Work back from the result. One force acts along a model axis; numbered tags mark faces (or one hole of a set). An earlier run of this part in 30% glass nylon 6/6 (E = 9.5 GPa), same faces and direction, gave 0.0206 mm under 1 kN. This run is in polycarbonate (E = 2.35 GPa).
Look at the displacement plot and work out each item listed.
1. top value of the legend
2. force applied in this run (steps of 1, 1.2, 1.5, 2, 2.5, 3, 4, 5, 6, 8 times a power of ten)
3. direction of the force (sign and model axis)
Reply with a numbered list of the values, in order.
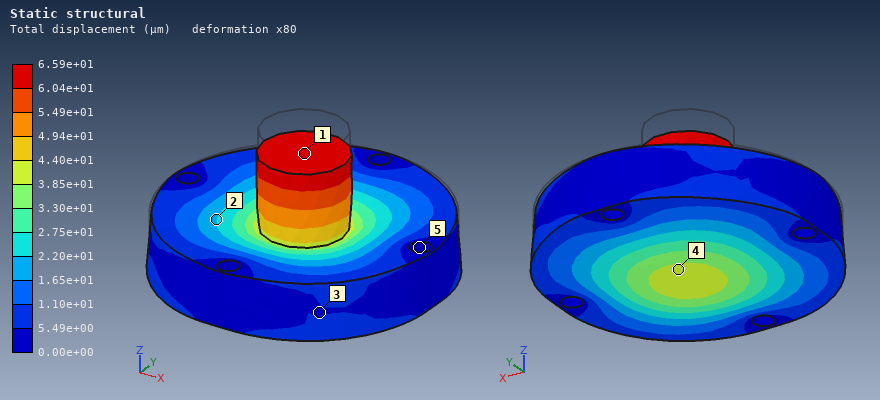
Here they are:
1. 6.59e+01 µm
2. 800 N
3. -Z
